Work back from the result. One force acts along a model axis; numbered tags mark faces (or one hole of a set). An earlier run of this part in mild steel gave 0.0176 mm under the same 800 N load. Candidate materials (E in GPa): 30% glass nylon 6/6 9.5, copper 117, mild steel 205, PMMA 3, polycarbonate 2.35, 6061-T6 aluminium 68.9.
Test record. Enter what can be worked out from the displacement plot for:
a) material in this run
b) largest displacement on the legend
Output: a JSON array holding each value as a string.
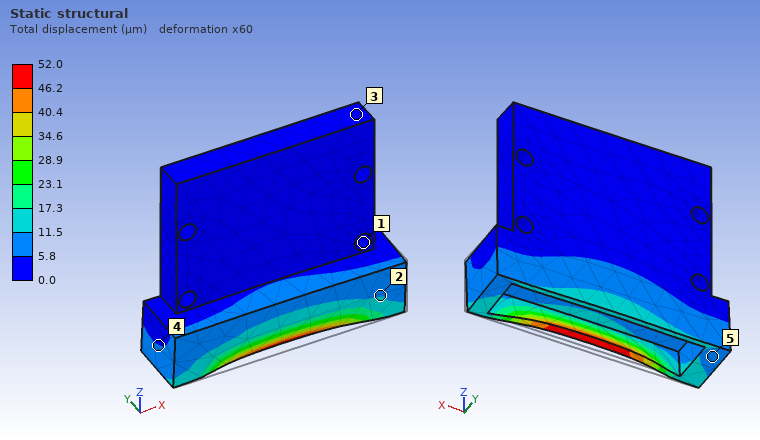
["6061-T6 aluminium", "52.0 µm"]
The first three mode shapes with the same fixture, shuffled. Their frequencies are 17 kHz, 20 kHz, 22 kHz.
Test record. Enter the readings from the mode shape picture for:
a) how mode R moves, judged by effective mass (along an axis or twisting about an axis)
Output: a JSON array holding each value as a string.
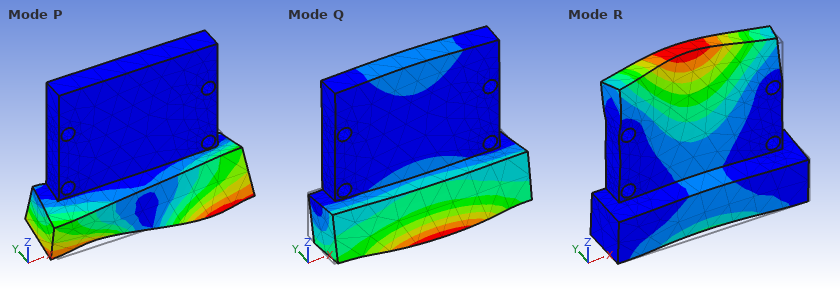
["along Y"]
